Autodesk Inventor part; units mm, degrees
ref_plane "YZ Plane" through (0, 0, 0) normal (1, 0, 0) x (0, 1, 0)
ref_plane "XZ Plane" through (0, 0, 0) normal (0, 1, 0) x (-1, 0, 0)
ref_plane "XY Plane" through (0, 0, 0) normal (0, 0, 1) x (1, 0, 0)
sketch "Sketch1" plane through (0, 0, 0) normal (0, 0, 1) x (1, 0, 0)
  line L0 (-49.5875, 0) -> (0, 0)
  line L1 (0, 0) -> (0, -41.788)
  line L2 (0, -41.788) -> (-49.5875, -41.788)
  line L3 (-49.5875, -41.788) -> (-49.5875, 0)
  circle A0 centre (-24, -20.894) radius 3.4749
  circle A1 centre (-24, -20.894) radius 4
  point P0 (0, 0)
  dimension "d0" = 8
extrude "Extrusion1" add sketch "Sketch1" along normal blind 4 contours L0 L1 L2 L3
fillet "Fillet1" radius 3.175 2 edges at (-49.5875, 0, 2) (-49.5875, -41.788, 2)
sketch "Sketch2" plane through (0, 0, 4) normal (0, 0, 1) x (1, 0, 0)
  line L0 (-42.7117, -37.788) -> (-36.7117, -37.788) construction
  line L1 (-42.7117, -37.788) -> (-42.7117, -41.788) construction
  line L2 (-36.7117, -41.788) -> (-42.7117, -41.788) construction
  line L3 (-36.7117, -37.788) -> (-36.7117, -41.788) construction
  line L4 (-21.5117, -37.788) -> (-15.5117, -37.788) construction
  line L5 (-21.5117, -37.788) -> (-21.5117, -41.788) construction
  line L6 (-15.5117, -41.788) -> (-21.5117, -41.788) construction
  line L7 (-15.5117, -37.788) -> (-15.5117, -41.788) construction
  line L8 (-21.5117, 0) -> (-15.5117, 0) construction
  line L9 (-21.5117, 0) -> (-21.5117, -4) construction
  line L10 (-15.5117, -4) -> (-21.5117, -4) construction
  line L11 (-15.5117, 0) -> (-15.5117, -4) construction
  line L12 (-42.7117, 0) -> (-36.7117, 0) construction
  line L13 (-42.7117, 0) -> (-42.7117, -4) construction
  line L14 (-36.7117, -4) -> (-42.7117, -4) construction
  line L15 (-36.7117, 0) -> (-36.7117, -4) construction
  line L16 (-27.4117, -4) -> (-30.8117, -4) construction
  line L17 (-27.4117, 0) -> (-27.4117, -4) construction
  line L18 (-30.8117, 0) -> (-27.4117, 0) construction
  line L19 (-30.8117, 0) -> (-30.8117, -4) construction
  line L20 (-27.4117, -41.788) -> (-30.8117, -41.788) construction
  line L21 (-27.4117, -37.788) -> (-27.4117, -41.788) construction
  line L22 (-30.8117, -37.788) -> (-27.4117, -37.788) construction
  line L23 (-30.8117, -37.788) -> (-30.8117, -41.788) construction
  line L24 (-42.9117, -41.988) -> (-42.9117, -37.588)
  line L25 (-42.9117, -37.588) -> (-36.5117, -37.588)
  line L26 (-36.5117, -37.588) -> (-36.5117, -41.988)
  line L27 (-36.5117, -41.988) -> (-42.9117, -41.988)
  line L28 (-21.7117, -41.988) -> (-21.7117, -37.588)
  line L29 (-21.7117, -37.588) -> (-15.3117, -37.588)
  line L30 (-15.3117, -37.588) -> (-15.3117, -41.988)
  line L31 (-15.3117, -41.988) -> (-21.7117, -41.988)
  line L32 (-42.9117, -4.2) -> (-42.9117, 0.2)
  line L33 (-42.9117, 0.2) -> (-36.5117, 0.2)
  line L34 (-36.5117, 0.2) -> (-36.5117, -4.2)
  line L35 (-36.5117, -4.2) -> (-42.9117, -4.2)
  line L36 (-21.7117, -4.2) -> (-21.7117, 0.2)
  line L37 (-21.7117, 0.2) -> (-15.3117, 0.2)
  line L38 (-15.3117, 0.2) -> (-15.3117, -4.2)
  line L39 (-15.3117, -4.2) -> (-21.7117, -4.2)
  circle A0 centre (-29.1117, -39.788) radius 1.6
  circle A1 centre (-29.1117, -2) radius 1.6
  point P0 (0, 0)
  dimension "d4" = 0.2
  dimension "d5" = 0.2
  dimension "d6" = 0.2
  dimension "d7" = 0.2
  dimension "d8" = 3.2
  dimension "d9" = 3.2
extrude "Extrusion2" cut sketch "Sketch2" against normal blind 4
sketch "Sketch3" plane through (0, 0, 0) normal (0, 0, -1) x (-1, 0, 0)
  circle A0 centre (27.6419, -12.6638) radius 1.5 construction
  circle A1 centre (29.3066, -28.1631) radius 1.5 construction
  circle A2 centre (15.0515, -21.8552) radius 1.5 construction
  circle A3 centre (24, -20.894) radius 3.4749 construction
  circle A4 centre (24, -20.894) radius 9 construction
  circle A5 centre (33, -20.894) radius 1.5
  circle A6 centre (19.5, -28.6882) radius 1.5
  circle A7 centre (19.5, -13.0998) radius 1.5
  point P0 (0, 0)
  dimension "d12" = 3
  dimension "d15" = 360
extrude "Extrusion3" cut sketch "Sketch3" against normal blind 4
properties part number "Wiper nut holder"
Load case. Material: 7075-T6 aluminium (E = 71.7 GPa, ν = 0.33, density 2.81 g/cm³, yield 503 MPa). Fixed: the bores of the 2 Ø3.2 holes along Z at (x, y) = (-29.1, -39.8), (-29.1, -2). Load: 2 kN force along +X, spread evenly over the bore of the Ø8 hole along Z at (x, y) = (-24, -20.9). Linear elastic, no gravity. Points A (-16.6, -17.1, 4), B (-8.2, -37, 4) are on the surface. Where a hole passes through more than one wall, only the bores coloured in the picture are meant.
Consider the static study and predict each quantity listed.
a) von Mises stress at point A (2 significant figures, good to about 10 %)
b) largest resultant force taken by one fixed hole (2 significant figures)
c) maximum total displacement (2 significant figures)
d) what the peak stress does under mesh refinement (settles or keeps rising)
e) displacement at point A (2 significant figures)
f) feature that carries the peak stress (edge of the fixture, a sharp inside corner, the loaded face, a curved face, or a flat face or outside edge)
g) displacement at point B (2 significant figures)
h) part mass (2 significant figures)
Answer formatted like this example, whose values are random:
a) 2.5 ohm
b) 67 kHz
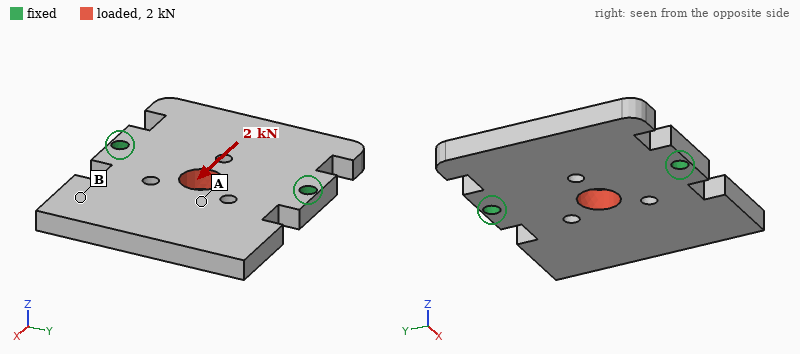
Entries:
a) 15 MPa
b) 1.0 kN
c) 9.5 µm
d) keeps rising
e) 7.4 µm
f) edge of the fixture
g) 5.7 µm
h) 21 g
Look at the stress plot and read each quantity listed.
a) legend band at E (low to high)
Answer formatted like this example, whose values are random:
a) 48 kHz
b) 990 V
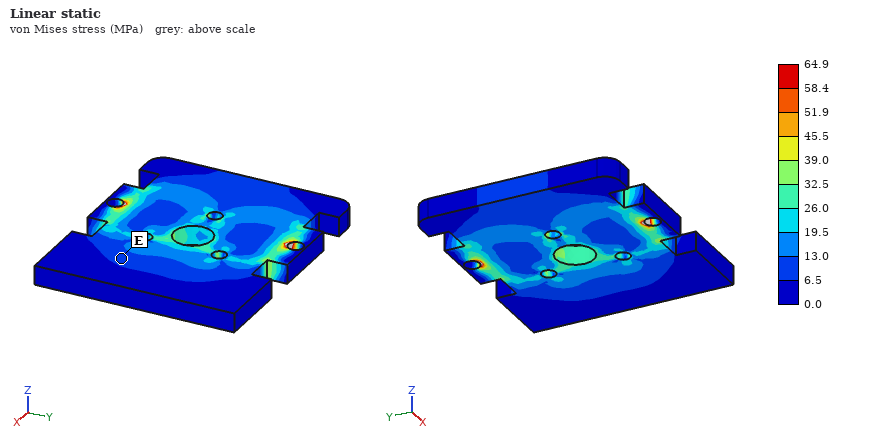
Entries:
a) 6.5 to 13.0 MPa
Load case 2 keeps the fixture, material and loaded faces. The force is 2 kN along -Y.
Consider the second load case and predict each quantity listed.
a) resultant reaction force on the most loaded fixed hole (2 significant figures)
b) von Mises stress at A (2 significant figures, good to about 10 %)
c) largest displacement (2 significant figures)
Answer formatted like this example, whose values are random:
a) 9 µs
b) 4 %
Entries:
a) 1.0 kN
b) 6.1 MPa
c) 7.9 µm
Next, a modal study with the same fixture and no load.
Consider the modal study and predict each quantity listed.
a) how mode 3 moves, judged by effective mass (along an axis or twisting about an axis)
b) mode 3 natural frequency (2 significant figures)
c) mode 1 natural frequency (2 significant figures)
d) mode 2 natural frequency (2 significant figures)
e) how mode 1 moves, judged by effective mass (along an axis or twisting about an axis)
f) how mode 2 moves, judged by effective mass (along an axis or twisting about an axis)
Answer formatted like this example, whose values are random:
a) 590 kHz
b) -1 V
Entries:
a) twisting about X
b) 6100 Hz
c) 2700 Hz
d) 5600 Hz
e) along Z
f) along Z
